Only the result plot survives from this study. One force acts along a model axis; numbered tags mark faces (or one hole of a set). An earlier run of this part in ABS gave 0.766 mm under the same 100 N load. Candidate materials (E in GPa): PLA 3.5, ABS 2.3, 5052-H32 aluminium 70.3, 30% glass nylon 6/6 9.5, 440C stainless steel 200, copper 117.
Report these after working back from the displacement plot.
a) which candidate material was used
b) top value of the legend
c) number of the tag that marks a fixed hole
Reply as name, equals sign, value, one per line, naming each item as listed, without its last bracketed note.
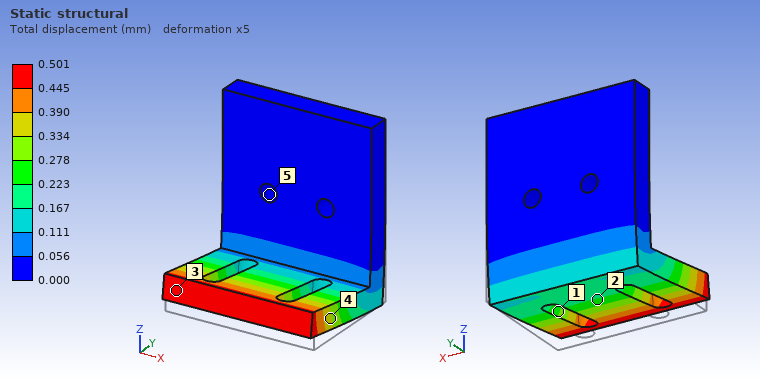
which candidate material was used = PLA
top value of the legend = 0.501 mm
number of the tag that marks a fixed hole = 5
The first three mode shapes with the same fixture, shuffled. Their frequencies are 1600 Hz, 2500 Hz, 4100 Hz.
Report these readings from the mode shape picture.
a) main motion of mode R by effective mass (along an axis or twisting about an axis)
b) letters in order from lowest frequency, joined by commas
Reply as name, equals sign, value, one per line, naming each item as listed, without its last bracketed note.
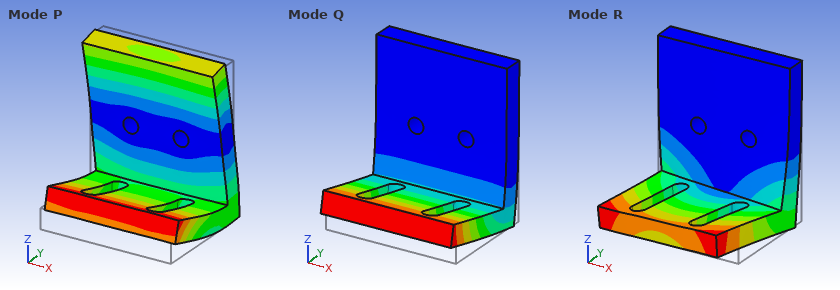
main motion of mode R by effective mass = along X
letters in order from lowest frequency, joined by commas = Q, R, P
